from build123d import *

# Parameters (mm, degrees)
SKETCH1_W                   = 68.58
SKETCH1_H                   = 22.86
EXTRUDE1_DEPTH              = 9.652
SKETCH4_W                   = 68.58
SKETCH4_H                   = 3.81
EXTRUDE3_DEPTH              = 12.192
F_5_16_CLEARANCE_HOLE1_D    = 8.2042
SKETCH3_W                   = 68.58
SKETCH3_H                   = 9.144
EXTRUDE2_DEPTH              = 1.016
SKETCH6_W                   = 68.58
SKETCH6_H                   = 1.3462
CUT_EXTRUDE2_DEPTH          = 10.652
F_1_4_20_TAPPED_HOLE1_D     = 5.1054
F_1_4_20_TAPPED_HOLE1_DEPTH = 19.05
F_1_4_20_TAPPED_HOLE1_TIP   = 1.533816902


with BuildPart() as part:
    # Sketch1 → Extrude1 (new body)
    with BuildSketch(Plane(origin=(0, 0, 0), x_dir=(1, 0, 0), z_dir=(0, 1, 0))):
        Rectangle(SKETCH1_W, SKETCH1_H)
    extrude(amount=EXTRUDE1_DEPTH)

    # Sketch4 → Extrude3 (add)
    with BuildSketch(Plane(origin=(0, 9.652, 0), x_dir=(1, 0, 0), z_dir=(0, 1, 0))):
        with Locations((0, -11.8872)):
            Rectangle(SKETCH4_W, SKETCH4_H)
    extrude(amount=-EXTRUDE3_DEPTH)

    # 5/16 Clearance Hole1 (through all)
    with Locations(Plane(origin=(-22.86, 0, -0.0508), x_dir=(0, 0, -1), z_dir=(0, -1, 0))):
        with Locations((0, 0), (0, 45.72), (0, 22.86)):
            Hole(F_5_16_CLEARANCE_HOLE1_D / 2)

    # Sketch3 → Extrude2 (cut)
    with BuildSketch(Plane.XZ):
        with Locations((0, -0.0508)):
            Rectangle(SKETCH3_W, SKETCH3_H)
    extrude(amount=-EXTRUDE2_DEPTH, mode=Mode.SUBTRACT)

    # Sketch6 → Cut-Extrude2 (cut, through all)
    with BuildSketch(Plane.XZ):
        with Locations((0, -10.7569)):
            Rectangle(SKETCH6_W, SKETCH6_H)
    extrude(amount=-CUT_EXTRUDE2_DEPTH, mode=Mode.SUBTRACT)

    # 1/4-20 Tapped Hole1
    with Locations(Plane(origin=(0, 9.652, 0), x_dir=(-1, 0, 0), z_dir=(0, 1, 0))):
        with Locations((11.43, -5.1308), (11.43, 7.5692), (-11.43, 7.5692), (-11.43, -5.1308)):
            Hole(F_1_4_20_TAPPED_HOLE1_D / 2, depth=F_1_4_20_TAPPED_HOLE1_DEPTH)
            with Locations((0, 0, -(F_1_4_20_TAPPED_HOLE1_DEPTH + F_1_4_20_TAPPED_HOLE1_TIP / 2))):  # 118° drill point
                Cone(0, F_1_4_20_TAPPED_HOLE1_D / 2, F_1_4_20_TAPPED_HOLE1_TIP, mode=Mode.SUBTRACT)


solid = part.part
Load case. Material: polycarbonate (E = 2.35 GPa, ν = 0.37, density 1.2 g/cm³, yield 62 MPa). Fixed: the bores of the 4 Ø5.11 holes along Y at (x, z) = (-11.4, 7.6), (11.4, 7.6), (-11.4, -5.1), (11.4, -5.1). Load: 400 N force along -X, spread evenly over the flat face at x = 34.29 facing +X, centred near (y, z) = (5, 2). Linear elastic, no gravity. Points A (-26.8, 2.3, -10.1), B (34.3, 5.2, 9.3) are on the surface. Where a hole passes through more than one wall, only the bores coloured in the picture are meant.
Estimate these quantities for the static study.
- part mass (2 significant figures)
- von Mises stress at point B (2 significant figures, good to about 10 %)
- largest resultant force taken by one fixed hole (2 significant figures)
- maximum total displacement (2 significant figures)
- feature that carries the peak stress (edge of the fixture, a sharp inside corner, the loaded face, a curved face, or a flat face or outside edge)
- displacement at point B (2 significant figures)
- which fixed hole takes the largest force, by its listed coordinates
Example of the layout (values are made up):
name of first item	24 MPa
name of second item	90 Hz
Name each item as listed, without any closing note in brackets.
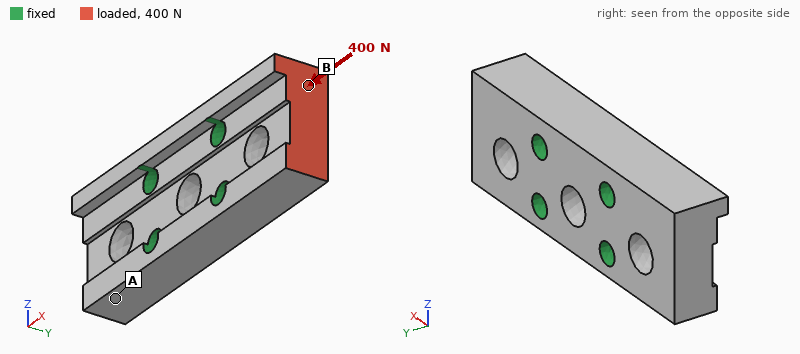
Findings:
part mass	16 g
von Mises stress at point B	1.8 MPa
largest resultant force taken by one fixed hole	220 N
maximum total displacement	27 µm
feature that carries the peak stress	a curved face
displacement at point B	19 µm
which fixed hole takes the largest force, by its listed coordinates	(11.4, 7.6)
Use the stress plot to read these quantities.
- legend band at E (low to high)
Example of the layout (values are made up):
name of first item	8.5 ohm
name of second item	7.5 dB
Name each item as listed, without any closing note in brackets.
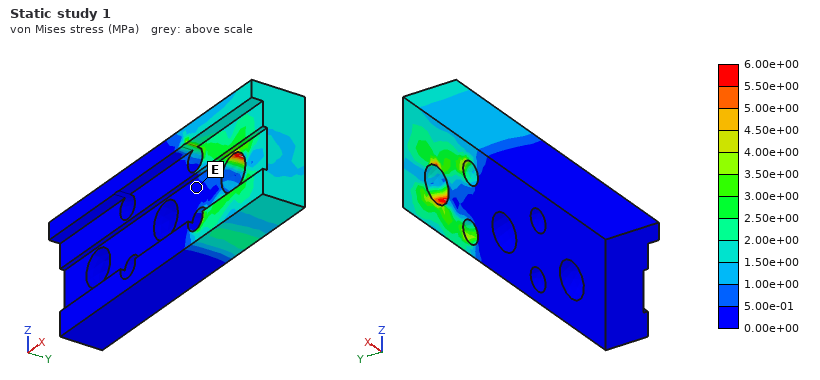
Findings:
legend band at E	0.00e+00 to 5.00e-01 MPa
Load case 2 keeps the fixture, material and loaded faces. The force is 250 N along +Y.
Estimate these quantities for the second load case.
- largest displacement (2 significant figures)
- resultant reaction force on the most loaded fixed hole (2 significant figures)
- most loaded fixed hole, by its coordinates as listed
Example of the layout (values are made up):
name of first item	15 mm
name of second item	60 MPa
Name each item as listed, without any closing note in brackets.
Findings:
largest displacement	0.29 mm
resultant reaction force on the most loaded fixed hole	160 N
most loaded fixed hole, by its coordinates as listed	(11.4, 7.6)
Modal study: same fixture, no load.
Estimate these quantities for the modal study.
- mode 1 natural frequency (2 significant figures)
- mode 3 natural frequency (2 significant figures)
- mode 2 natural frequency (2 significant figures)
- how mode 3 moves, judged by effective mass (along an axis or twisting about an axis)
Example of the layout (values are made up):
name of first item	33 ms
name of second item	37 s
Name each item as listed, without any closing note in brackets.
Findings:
mode 1 natural frequency	4000 Hz
mode 3 natural frequency	5500 Hz
mode 2 natural frequency	4000 Hz
how mode 3 moves, judged by effective mass	twisting about Y
